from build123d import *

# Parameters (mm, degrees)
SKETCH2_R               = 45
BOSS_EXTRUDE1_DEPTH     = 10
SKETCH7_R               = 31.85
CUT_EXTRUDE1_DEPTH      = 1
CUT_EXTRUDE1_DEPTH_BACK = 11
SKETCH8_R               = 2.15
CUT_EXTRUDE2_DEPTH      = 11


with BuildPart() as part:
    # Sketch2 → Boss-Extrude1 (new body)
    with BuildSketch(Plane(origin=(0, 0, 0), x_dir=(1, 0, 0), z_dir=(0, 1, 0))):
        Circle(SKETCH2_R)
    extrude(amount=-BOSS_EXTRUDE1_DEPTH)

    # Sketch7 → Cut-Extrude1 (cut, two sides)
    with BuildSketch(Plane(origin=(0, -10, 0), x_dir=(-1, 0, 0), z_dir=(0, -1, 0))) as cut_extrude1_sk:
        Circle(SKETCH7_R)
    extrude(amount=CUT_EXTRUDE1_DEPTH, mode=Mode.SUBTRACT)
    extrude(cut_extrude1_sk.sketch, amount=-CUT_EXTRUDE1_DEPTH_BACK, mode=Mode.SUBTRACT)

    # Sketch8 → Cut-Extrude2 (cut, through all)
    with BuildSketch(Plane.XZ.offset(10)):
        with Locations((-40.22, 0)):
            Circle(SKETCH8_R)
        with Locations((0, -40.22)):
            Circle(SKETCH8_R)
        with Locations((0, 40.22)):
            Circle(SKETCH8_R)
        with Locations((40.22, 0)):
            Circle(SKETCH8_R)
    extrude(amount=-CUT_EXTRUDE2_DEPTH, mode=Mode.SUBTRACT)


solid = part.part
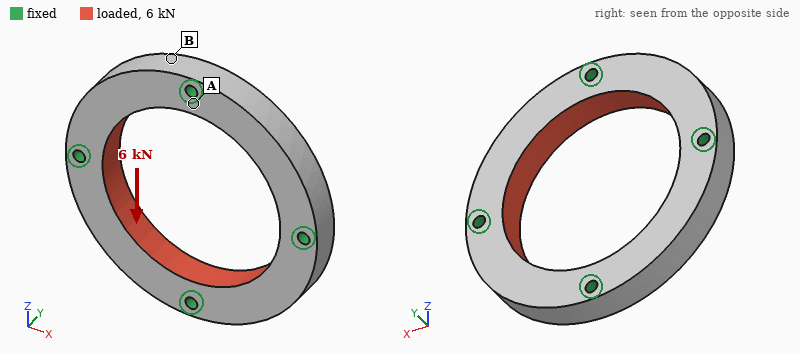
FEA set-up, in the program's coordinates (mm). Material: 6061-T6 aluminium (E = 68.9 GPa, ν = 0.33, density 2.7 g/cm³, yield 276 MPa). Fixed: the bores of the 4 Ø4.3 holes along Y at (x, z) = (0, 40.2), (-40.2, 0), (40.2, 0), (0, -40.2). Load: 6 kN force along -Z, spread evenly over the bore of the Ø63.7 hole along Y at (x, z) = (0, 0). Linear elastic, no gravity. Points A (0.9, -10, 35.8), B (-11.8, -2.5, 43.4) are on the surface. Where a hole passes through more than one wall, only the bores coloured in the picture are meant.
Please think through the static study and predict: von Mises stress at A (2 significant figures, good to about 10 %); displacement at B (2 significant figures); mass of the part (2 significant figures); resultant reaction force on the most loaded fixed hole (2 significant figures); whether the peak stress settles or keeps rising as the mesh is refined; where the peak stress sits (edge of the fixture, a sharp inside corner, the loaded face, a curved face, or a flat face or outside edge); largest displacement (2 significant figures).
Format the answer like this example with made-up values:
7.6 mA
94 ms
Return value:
10 MPa
2.5 µm
84 g
2.0 kN
keeps rising
edge of the fixture
5.3 µm
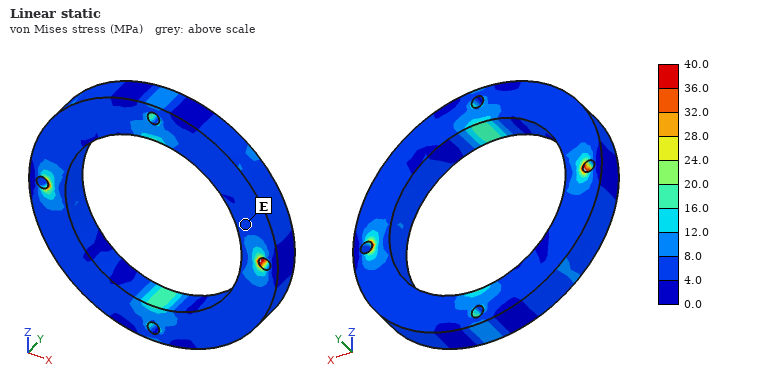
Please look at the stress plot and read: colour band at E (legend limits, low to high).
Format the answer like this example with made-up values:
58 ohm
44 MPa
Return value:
4.0 to 8.0 MPa
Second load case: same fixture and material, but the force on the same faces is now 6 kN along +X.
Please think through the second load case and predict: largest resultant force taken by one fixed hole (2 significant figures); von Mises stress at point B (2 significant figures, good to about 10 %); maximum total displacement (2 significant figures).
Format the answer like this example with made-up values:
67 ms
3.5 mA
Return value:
2.0 kN
5.6 MPa
5.3 µm
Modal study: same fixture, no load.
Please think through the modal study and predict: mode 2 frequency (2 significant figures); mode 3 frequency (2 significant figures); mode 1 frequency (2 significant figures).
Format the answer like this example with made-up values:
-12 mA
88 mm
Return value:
11 kHz
11 kHz
11 kHz
